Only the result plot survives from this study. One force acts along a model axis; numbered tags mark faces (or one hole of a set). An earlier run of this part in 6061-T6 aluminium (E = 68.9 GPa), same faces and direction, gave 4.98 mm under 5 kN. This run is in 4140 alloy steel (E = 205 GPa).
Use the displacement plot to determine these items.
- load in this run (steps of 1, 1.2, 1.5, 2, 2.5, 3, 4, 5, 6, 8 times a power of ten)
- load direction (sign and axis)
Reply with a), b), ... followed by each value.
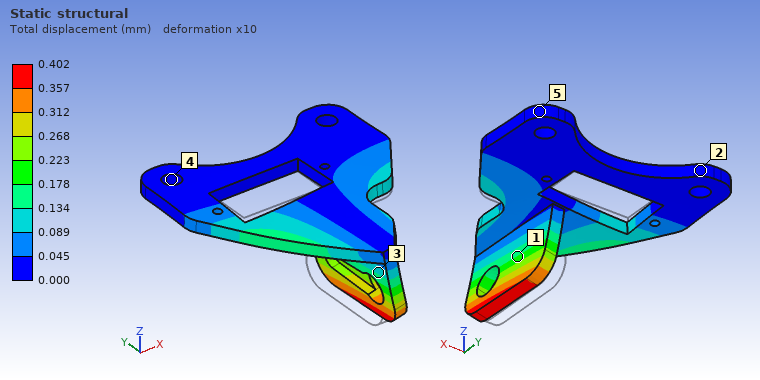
a) 1.2 kN
b) +X
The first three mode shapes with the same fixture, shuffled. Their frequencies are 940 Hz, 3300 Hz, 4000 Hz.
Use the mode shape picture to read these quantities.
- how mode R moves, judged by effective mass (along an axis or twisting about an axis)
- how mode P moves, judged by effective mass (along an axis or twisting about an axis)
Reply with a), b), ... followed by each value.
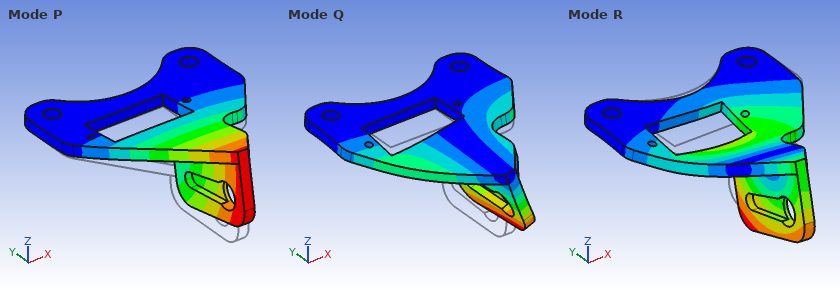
a) along Z
b) along Z
